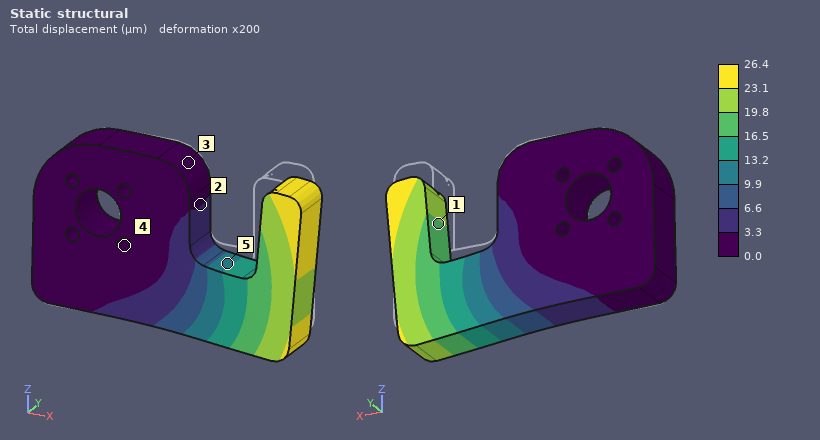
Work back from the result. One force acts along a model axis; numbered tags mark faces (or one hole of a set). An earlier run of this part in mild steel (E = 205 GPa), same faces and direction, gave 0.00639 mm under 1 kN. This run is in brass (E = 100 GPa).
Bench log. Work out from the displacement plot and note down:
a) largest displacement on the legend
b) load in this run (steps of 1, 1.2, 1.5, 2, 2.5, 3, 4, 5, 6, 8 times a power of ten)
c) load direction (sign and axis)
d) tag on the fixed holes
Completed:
26.4 µm
2 kN
-Z
4
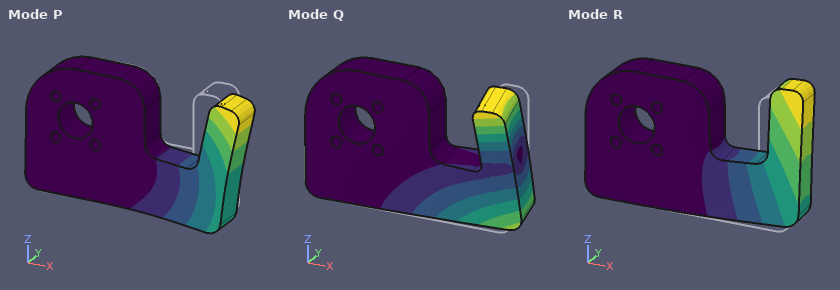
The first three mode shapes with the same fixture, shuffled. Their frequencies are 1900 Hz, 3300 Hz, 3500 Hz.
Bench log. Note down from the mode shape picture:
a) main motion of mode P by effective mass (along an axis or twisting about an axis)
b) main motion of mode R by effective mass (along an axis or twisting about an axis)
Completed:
along Z
along Y
